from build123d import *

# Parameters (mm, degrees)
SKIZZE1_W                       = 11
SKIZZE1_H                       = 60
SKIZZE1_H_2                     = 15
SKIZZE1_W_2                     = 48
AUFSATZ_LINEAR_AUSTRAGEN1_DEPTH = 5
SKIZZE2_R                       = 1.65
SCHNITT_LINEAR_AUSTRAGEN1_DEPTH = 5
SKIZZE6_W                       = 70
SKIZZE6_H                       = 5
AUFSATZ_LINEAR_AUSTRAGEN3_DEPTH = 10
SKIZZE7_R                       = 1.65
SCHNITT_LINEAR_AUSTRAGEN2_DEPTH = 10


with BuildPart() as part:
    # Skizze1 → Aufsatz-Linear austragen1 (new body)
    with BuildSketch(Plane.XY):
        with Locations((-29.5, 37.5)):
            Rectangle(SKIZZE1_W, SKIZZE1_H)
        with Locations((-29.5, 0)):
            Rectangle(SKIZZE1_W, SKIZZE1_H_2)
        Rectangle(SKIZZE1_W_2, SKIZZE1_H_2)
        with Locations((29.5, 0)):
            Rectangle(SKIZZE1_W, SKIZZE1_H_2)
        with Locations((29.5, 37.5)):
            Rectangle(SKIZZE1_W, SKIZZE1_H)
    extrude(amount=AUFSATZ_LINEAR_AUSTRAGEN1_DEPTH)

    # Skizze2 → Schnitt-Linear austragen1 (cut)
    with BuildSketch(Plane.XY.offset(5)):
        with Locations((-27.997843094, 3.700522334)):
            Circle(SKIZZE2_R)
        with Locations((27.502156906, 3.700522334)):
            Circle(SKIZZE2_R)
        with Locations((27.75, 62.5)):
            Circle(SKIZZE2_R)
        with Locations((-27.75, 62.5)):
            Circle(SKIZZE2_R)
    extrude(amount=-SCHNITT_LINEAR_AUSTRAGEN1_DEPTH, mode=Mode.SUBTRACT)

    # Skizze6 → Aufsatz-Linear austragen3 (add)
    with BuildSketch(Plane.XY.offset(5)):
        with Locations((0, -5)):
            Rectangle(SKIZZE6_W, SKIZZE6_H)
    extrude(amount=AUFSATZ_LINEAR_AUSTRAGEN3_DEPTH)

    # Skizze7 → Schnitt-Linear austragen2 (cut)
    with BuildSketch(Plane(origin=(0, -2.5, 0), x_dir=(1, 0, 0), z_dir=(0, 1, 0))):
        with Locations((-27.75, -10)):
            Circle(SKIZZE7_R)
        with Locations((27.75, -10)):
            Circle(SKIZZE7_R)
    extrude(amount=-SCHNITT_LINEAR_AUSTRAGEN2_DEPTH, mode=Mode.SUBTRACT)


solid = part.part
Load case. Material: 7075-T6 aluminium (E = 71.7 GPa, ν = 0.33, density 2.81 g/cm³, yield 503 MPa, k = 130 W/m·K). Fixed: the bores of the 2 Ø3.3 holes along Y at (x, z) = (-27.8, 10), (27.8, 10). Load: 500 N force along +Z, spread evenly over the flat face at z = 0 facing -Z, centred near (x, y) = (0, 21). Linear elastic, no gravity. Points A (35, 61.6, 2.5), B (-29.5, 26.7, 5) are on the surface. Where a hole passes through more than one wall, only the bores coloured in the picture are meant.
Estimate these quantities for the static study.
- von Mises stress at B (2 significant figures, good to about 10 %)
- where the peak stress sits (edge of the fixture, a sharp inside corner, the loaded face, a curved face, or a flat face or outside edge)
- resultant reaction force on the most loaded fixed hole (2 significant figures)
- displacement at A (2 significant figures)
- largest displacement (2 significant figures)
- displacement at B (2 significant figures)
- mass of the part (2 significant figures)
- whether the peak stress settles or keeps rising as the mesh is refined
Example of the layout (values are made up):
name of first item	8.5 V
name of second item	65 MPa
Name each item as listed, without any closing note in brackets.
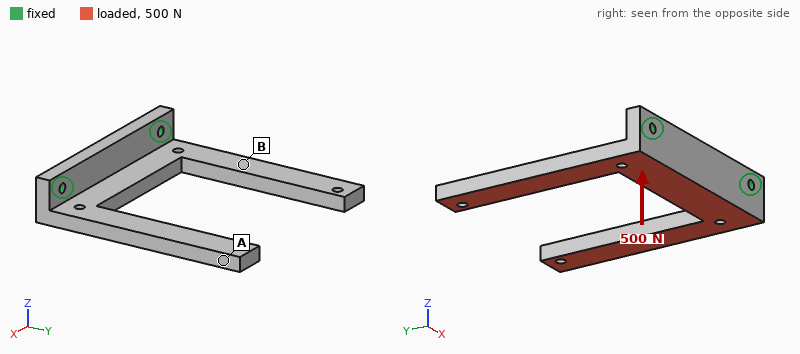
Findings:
von Mises stress at B	41 MPa
where the peak stress sits	edge of the fixture
resultant reaction force on the most loaded fixed hole	250 N
displacement at A	0.95 mm
largest displacement	1.1 mm
displacement at B	0.32 mm
mass of the part	42 g
whether the peak stress settles or keeps rising as the mesh is refined	keeps rising
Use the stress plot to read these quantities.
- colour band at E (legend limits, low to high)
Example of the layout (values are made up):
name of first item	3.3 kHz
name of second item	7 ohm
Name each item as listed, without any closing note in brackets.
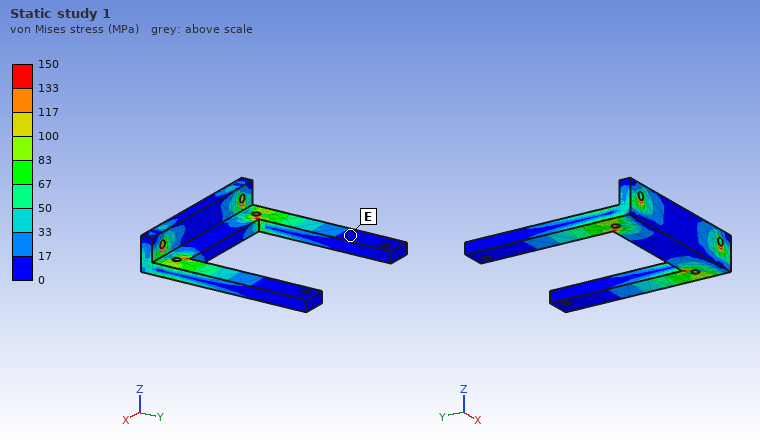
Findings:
colour band at E	0 to 17 MPa
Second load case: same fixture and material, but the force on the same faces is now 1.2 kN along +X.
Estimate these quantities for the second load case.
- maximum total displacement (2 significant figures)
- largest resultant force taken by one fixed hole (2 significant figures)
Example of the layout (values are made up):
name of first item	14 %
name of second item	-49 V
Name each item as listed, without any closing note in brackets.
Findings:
maximum total displacement	0.41 mm
largest resultant force taken by one fixed hole	790 N
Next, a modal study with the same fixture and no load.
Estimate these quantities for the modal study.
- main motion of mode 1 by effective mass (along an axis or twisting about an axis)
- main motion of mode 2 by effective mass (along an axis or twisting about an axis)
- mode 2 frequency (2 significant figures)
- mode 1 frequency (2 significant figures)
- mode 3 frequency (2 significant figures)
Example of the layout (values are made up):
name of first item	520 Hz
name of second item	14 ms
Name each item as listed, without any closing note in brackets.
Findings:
main motion of mode 1 by effective mass	along Z
main motion of mode 2 by effective mass	twisting about Y
mode 2 frequency	790 Hz
mode 1 frequency	760 Hz
mode 3 frequency	1800 Hz
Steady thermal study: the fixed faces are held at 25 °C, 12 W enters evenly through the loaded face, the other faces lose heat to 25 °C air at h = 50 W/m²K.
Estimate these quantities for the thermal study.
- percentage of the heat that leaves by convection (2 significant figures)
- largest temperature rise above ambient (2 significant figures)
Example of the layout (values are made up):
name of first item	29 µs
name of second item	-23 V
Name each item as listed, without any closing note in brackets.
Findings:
percentage of the heat that leaves by convection	20 %
largest temperature rise above ambient	16 K
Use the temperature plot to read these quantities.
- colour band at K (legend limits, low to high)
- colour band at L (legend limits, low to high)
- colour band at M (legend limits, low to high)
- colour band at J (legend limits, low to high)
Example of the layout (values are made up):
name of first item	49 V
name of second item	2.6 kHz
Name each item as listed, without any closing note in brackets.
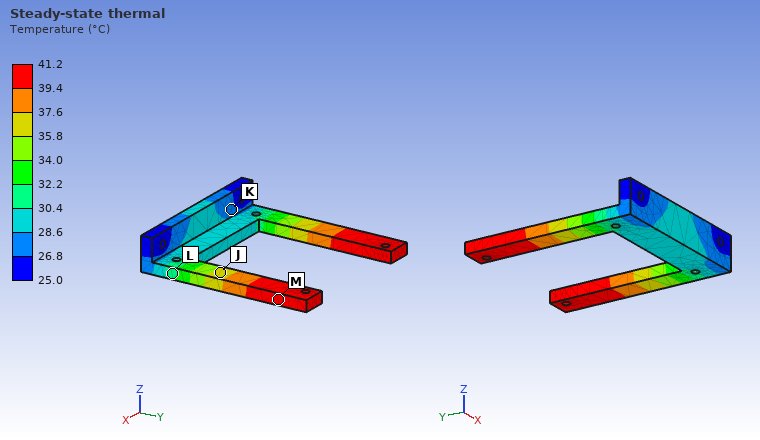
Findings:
colour band at K	26.8 to 28.6 °C
colour band at L	30.4 to 32.2 °C
colour band at M	39.4 to 41.2 °C
colour band at J	35.8 to 37.6 °C
